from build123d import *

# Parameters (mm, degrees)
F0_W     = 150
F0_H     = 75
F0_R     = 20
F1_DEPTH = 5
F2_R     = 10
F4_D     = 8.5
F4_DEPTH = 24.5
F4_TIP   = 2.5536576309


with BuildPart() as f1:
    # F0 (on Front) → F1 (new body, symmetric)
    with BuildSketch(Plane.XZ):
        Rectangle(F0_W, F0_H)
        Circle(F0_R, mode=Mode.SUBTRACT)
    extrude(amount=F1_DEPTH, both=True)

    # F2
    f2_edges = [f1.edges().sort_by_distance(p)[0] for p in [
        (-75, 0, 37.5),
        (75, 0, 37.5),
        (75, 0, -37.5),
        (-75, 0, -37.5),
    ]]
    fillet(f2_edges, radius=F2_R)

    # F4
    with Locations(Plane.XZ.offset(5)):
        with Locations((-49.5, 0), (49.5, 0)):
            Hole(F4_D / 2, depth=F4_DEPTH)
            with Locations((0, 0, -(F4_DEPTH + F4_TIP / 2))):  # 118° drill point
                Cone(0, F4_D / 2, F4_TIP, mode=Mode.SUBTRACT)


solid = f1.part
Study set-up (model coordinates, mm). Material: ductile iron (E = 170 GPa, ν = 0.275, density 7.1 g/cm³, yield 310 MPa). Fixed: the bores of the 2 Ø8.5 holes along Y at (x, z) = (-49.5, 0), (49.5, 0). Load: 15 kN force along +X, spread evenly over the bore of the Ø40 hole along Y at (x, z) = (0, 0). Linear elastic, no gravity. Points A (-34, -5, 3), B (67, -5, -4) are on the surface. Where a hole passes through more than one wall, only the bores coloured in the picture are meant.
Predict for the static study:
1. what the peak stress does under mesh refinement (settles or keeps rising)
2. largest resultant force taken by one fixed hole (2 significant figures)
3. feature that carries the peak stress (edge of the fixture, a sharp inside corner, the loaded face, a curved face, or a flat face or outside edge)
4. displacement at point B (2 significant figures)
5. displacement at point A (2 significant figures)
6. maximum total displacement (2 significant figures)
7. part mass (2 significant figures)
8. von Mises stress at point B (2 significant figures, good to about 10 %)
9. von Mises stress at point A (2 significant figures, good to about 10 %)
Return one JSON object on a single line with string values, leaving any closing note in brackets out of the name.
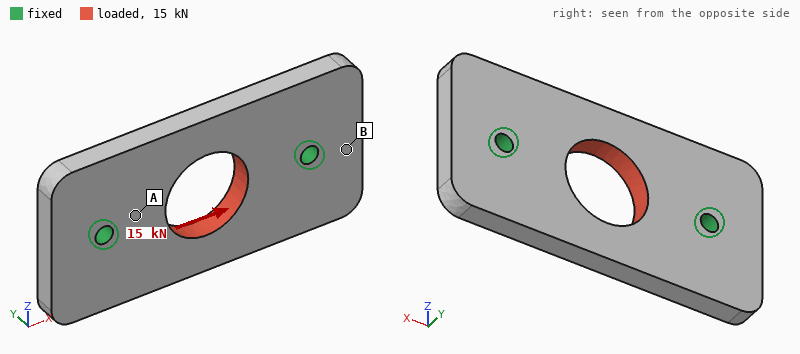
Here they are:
{"what the peak stress does under mesh refinement": "keeps rising", "largest resultant force taken by one fixed hole": "7.5 kN", "feature that carries the peak stress": "edge of the fixture", "displacement at point B": "0.86 µm", "displacement at point A": "1.9 µm", "maximum total displacement": "5.5 µm", "part mass": "700 g", "von Mises stress at point B": "7.9 MPa", "von Mises stress at point A": "22 MPa"}
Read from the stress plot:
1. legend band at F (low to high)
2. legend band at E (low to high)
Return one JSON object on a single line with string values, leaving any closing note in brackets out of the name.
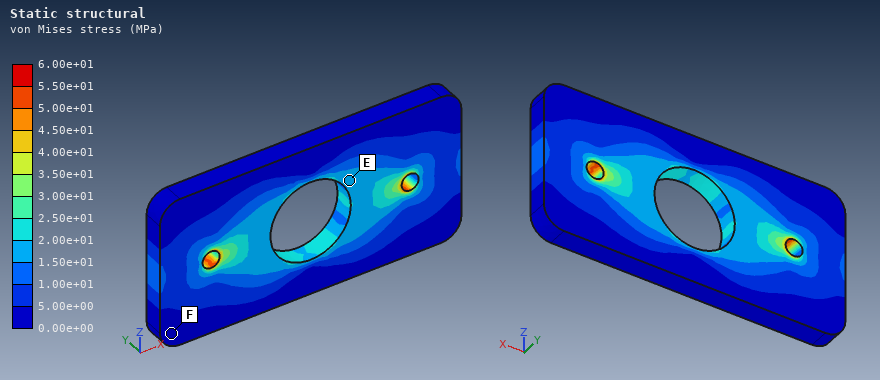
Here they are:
{"legend band at F": "0.00e+00 to 5.00e+00 MPa", "legend band at E": "1.50e+01 to 2.00e+01 MPa"}
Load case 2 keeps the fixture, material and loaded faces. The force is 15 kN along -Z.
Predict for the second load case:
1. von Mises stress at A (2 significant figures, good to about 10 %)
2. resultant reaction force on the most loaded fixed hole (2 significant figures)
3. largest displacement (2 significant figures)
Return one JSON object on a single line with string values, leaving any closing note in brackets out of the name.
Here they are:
{"von Mises stress at A": "26 MPa", "resultant reaction force on the most loaded fixed hole": "7.5 kN", "largest displacement": "13 µm"}
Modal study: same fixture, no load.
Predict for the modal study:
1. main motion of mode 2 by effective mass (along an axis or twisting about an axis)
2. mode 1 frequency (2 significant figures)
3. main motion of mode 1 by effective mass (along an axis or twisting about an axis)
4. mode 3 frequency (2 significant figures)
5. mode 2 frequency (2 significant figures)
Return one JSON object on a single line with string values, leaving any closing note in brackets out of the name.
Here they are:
{"main motion of mode 2 by effective mass": "along Y", "mode 1 frequency": "3300 Hz", "main motion of mode 1 by effective mass": "twisting about X", "mode 3 frequency": "5000 Hz", "mode 2 frequency": "3700 Hz"}
